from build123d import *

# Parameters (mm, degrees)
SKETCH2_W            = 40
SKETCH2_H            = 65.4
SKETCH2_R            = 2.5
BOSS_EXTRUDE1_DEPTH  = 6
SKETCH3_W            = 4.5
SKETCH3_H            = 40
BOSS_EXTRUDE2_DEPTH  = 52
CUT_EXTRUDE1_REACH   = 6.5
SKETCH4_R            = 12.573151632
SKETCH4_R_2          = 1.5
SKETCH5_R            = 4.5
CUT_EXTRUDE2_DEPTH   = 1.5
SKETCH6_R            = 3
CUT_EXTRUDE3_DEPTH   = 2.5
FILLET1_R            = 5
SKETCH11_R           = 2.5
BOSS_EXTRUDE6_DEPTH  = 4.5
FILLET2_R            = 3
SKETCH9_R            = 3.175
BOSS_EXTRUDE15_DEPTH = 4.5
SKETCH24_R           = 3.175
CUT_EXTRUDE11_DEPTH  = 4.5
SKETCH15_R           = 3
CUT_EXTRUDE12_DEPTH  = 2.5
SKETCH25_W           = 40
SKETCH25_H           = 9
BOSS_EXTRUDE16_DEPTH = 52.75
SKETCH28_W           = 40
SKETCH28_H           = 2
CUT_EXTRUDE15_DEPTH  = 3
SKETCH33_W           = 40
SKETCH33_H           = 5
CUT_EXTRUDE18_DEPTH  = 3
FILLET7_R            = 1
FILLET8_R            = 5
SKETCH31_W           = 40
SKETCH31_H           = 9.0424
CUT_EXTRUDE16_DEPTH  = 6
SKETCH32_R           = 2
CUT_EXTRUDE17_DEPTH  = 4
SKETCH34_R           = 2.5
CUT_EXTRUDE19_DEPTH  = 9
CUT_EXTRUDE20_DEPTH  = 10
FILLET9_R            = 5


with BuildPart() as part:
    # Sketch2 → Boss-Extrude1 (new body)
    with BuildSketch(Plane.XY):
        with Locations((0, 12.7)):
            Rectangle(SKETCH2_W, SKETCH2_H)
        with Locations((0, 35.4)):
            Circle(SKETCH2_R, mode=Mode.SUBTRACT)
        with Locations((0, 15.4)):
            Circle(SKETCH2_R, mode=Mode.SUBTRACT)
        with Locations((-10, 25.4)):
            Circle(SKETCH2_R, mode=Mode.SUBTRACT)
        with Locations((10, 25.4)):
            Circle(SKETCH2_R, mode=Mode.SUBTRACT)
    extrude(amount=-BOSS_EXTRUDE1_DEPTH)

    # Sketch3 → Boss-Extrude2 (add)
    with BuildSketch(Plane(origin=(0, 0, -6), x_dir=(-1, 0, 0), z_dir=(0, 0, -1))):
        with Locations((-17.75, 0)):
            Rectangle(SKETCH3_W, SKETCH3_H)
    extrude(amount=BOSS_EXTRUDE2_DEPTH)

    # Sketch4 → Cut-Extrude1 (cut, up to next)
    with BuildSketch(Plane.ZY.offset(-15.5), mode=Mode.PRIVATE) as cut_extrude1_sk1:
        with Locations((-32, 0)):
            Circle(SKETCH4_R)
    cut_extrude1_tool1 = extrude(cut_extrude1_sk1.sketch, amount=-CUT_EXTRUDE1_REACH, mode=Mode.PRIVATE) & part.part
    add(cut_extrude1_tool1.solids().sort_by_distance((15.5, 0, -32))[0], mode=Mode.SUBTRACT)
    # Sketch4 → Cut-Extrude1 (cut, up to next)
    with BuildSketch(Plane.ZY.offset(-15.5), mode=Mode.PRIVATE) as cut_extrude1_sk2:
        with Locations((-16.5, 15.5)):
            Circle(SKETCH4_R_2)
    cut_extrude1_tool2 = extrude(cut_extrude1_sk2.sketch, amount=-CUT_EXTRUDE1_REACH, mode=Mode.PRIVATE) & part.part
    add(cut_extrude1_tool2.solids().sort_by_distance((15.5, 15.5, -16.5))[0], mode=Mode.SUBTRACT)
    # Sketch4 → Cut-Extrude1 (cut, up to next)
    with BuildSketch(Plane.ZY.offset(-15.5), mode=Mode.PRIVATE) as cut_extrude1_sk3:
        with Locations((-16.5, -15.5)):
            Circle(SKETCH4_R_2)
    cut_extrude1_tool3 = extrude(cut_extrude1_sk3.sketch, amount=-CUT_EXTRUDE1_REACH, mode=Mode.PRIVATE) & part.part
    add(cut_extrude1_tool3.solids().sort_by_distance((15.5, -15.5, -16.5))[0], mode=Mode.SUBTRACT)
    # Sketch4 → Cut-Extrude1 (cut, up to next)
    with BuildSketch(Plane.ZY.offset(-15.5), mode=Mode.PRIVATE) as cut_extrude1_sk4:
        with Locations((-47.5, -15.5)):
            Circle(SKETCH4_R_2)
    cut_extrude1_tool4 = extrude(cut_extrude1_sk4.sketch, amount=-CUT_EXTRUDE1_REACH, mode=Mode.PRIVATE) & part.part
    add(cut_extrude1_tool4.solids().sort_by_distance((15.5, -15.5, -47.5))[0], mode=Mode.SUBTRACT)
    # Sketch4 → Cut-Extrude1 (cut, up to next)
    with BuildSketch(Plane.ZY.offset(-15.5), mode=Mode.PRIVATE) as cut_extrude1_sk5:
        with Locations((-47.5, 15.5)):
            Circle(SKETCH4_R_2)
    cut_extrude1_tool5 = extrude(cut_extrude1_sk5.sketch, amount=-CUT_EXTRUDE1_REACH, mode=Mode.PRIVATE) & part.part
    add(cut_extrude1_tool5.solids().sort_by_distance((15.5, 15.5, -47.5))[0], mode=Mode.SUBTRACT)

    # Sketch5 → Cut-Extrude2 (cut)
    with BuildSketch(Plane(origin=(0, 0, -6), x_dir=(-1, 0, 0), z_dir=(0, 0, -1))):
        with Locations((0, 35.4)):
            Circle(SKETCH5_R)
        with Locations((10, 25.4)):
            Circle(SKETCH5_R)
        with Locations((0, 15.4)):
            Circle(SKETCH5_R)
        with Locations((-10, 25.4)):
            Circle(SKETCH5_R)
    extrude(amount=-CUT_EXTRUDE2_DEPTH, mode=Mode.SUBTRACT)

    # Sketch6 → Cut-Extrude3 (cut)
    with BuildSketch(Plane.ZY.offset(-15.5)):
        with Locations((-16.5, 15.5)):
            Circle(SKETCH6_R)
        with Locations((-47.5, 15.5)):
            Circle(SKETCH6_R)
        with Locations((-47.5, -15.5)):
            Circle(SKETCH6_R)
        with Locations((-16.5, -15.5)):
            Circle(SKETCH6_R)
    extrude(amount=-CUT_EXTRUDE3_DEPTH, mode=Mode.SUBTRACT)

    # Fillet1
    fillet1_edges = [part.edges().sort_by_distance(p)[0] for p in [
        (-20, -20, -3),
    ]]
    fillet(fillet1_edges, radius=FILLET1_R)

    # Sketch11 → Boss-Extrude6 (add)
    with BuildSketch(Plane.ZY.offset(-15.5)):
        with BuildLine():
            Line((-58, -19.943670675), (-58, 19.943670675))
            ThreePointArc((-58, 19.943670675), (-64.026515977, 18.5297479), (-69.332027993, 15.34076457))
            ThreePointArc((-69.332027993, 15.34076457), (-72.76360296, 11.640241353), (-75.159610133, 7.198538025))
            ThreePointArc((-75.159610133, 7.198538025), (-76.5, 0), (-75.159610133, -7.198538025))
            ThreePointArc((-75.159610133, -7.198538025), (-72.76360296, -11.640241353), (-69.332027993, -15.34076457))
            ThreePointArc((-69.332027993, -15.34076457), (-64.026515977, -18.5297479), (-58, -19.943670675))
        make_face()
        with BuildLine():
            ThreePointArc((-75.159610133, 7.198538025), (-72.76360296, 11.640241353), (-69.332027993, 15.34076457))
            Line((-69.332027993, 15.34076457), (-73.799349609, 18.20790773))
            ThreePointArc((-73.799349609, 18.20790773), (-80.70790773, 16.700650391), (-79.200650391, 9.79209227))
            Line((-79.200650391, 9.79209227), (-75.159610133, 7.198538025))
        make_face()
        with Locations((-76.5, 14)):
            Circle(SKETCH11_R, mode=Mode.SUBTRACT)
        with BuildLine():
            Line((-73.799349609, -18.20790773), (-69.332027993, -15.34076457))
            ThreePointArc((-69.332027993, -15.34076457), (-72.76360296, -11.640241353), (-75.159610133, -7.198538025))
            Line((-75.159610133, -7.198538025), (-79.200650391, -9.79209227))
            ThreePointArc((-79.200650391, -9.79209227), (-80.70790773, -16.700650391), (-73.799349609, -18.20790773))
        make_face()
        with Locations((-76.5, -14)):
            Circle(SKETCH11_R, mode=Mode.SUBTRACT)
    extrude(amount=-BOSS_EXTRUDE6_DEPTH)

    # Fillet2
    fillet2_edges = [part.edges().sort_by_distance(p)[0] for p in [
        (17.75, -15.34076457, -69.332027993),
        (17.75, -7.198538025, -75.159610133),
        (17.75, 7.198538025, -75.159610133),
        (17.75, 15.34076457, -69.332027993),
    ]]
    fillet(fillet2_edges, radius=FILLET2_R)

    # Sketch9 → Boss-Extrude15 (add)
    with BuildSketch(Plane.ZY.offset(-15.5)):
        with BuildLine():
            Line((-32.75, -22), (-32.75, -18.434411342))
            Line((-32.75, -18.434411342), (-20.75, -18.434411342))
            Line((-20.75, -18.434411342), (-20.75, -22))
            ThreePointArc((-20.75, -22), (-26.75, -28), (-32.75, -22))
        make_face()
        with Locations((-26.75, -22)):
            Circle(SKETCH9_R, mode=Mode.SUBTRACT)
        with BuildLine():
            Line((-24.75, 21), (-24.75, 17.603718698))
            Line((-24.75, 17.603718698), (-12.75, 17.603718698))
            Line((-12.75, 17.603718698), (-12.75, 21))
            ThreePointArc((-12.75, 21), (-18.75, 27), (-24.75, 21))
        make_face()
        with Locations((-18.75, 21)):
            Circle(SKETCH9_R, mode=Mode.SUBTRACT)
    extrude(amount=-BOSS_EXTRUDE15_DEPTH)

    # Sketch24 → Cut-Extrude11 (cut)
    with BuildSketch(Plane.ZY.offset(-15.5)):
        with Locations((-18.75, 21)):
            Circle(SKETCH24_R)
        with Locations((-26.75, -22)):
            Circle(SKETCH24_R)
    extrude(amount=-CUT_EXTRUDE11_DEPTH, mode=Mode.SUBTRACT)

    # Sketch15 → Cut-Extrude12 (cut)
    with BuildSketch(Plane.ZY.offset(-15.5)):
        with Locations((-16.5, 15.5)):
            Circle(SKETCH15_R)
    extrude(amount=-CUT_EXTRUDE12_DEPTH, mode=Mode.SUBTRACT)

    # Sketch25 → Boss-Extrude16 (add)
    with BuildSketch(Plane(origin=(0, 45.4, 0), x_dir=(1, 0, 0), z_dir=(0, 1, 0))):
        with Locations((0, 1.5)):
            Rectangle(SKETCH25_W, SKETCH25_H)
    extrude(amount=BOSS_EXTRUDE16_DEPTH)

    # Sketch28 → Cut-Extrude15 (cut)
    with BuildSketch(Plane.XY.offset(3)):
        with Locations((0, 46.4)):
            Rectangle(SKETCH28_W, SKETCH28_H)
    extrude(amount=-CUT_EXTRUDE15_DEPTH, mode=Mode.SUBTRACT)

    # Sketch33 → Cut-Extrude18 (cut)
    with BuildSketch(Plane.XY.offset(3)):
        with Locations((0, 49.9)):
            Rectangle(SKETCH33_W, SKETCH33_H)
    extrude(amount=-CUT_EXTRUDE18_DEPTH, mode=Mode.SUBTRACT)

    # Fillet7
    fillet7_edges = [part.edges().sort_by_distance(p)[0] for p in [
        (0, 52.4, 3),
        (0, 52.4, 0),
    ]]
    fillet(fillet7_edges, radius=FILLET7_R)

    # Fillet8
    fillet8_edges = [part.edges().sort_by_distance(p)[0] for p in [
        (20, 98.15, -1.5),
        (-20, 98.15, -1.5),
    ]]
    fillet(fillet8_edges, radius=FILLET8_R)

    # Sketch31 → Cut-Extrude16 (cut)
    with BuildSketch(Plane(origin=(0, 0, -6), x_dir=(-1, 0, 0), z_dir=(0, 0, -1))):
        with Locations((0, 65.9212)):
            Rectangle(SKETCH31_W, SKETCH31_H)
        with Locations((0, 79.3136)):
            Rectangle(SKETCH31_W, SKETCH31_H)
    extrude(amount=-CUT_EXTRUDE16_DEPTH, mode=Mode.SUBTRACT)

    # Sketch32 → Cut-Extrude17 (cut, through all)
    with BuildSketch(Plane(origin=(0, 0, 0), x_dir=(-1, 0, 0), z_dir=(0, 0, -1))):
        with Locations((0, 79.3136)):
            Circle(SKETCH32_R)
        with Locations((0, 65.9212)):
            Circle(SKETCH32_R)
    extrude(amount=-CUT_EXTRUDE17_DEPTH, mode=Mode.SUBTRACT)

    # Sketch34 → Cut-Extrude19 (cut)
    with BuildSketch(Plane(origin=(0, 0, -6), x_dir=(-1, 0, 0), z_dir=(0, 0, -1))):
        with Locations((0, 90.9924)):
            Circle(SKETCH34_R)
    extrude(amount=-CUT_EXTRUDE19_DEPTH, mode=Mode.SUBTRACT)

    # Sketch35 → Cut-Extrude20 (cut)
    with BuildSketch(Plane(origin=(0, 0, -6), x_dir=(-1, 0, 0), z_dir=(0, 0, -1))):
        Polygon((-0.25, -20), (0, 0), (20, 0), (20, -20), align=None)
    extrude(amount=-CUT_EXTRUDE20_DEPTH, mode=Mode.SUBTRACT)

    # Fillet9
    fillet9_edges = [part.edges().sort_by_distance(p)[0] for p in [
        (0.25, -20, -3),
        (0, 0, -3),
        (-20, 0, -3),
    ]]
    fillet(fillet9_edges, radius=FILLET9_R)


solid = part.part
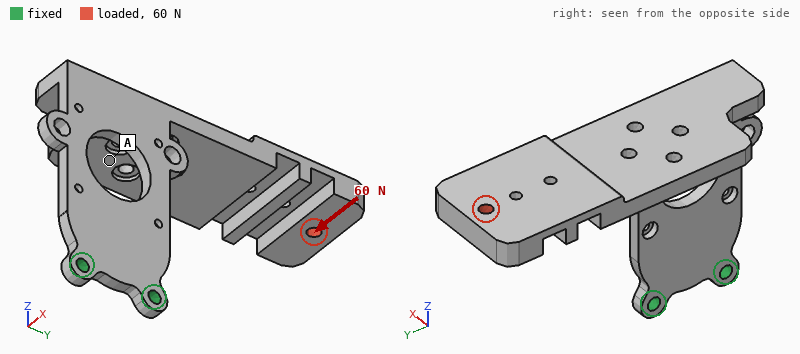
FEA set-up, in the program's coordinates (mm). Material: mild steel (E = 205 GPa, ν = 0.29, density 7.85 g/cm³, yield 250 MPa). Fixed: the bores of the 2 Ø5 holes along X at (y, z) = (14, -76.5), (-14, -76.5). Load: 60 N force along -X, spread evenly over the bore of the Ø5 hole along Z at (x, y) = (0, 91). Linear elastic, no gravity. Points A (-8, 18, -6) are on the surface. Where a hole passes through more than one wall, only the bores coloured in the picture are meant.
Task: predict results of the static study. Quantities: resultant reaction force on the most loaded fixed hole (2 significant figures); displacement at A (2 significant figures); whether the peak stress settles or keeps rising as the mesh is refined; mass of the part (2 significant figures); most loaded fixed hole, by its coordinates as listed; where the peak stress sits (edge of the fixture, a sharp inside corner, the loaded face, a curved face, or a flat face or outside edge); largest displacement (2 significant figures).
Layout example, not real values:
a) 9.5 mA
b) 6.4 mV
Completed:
a) 220 N
b) 0.33 mm
c) keeps rising
d) 290 g
e) (14, -76.5)
f) edge of the fixture
g) 0.79 mm
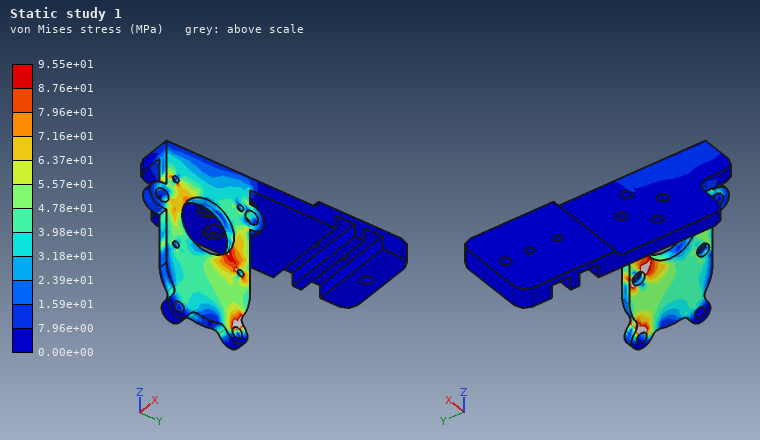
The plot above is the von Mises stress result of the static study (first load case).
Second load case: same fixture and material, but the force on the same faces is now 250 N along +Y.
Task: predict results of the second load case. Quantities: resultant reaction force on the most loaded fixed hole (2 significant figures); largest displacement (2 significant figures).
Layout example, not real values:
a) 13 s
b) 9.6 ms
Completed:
a) 710 N
b) 0.45 mm
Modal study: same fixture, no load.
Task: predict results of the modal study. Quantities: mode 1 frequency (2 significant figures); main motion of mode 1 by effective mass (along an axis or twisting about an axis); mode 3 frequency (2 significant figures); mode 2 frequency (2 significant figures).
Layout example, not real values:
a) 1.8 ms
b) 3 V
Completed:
a) 140 Hz
b) along X
c) 470 Hz
d) 300 Hz
